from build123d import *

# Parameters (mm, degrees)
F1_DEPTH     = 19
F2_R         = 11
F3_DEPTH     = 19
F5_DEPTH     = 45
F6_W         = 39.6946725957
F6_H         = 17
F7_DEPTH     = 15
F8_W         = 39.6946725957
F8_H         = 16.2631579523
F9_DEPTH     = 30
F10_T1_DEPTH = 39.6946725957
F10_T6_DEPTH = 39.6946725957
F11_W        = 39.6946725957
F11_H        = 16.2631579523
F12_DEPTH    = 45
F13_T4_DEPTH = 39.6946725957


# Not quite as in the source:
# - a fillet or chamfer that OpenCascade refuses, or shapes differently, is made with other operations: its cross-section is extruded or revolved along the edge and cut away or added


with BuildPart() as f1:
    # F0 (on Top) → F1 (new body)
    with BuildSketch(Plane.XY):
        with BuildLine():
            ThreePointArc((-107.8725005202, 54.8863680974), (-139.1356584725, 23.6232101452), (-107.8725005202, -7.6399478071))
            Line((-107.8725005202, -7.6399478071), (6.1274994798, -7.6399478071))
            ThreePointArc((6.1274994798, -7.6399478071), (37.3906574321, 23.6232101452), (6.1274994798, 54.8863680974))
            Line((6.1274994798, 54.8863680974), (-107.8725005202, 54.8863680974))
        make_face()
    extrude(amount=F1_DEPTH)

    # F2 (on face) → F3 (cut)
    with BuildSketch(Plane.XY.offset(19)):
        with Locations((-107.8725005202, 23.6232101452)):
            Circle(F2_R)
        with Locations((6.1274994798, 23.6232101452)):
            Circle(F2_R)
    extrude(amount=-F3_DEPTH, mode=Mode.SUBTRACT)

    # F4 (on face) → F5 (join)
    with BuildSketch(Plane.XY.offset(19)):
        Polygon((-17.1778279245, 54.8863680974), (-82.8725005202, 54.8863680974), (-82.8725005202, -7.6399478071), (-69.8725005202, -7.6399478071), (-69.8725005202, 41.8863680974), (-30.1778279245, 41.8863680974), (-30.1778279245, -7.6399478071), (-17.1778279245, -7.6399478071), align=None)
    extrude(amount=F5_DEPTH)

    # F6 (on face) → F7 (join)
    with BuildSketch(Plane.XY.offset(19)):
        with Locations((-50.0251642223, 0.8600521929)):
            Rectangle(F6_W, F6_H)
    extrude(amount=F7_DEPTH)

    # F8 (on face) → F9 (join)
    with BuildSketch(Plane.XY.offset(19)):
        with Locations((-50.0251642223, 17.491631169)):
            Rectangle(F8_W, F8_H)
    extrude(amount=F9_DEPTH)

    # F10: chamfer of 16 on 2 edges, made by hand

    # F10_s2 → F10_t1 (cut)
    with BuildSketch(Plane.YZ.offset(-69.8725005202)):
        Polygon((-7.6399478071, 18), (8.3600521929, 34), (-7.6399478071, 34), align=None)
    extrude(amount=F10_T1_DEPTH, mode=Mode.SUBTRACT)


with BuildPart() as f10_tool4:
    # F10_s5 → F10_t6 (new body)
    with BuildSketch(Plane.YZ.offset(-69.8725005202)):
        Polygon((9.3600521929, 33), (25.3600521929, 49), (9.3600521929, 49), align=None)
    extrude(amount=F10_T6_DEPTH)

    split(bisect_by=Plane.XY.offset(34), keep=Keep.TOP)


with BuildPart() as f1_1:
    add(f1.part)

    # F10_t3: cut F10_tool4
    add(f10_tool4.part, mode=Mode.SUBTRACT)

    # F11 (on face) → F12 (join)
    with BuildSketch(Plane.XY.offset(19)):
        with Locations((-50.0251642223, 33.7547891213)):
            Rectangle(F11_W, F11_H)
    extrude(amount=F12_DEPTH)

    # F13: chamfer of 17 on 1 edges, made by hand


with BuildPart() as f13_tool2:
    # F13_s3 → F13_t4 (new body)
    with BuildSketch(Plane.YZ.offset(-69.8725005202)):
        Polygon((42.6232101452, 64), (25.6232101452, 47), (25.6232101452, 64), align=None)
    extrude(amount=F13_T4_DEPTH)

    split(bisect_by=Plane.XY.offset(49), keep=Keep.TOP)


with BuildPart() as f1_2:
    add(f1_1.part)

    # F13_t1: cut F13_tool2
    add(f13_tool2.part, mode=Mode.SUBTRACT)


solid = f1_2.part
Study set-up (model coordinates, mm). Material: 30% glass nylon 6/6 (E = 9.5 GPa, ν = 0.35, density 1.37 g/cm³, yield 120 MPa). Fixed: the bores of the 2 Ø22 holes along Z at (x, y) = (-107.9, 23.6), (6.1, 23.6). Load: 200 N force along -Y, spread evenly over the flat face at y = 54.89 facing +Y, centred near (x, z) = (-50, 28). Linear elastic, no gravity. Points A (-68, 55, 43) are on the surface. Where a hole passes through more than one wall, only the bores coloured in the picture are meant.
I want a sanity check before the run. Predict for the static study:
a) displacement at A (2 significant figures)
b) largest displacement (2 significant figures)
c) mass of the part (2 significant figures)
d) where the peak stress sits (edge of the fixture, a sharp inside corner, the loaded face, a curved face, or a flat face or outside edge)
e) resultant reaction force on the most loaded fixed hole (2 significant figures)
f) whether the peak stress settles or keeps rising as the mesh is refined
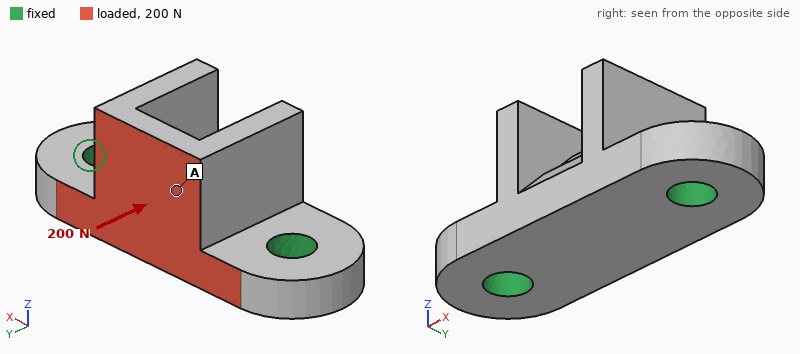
4.8 µm
6.5 µm
440 g
edge of the fixture
100 N
keeps rising
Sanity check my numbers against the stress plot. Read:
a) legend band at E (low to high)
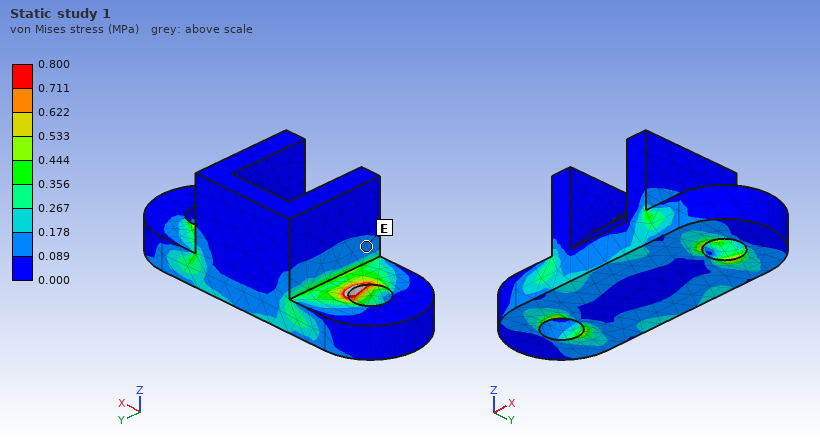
0.089 to 0.178 MPa
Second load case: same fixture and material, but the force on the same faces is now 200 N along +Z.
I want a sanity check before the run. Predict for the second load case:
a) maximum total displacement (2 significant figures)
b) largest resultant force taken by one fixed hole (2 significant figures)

9.0 µm
110 N
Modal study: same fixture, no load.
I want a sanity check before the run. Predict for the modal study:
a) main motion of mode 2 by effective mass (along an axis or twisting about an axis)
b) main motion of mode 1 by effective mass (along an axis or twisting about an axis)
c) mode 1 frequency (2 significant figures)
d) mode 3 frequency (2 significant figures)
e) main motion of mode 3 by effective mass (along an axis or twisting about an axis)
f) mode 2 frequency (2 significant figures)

along Z
along Y
1800 Hz
3800 Hz
along X
3300 Hz
